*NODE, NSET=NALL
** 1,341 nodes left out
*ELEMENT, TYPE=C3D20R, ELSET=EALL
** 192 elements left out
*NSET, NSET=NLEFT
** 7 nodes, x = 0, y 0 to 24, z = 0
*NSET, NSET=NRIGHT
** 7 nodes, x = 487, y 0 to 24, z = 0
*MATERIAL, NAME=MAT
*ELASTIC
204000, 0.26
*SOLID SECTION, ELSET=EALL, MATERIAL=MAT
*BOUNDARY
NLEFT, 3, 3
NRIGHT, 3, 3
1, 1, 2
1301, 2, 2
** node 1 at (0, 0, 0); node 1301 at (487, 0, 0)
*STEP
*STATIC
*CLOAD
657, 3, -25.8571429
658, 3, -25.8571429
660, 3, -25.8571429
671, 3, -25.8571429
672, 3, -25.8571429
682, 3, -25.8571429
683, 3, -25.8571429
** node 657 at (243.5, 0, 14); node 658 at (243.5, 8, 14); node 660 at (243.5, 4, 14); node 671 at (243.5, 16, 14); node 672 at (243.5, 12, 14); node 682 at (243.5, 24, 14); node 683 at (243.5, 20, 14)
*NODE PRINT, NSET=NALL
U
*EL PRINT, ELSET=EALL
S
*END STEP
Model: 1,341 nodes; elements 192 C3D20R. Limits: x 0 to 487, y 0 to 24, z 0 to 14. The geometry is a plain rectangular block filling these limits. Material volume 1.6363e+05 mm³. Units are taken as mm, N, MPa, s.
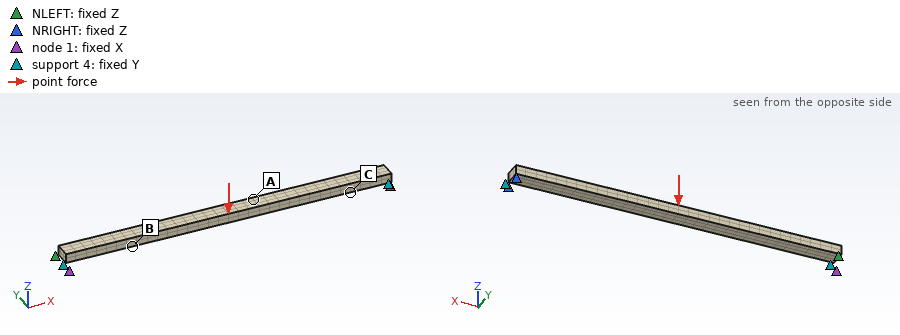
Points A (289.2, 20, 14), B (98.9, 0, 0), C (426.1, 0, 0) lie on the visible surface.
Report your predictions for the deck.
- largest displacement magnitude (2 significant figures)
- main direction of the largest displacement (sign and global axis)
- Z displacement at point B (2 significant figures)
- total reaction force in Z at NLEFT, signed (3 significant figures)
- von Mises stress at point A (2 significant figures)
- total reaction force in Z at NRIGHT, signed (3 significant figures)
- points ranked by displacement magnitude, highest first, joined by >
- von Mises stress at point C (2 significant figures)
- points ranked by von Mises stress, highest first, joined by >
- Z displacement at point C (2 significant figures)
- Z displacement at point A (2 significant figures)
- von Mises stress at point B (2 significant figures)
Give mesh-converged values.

0.39 mm
-Z
-0.22 mm
90.5 N
23 MPa
90.5 N
A > B > C
7.0 MPa
A > B > C
-0.14 mm
-0.37 mm
11 MPa
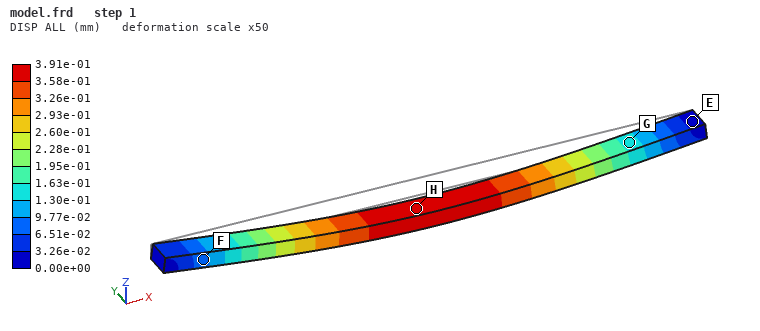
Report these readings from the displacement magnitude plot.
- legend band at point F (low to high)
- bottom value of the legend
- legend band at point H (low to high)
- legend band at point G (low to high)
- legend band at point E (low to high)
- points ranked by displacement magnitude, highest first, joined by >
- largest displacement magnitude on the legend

6.51e-02 to 9.77e-02 mm
0.00e+00 mm
3.58e-01 to 3.91e-01 mm
1.30e-01 to 1.63e-01 mm
0.00e+00 to 3.26e-02 mm
H > G > F > E
3.91e-01 mm
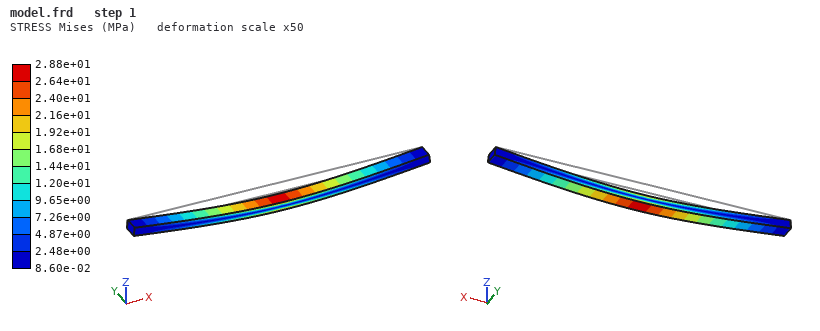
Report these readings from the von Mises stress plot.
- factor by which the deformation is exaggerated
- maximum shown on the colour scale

50
2.88e+01 MPa
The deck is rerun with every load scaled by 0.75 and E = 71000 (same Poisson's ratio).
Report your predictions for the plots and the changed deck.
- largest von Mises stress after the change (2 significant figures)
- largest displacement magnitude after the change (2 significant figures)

22 MPa
0.84 mm
